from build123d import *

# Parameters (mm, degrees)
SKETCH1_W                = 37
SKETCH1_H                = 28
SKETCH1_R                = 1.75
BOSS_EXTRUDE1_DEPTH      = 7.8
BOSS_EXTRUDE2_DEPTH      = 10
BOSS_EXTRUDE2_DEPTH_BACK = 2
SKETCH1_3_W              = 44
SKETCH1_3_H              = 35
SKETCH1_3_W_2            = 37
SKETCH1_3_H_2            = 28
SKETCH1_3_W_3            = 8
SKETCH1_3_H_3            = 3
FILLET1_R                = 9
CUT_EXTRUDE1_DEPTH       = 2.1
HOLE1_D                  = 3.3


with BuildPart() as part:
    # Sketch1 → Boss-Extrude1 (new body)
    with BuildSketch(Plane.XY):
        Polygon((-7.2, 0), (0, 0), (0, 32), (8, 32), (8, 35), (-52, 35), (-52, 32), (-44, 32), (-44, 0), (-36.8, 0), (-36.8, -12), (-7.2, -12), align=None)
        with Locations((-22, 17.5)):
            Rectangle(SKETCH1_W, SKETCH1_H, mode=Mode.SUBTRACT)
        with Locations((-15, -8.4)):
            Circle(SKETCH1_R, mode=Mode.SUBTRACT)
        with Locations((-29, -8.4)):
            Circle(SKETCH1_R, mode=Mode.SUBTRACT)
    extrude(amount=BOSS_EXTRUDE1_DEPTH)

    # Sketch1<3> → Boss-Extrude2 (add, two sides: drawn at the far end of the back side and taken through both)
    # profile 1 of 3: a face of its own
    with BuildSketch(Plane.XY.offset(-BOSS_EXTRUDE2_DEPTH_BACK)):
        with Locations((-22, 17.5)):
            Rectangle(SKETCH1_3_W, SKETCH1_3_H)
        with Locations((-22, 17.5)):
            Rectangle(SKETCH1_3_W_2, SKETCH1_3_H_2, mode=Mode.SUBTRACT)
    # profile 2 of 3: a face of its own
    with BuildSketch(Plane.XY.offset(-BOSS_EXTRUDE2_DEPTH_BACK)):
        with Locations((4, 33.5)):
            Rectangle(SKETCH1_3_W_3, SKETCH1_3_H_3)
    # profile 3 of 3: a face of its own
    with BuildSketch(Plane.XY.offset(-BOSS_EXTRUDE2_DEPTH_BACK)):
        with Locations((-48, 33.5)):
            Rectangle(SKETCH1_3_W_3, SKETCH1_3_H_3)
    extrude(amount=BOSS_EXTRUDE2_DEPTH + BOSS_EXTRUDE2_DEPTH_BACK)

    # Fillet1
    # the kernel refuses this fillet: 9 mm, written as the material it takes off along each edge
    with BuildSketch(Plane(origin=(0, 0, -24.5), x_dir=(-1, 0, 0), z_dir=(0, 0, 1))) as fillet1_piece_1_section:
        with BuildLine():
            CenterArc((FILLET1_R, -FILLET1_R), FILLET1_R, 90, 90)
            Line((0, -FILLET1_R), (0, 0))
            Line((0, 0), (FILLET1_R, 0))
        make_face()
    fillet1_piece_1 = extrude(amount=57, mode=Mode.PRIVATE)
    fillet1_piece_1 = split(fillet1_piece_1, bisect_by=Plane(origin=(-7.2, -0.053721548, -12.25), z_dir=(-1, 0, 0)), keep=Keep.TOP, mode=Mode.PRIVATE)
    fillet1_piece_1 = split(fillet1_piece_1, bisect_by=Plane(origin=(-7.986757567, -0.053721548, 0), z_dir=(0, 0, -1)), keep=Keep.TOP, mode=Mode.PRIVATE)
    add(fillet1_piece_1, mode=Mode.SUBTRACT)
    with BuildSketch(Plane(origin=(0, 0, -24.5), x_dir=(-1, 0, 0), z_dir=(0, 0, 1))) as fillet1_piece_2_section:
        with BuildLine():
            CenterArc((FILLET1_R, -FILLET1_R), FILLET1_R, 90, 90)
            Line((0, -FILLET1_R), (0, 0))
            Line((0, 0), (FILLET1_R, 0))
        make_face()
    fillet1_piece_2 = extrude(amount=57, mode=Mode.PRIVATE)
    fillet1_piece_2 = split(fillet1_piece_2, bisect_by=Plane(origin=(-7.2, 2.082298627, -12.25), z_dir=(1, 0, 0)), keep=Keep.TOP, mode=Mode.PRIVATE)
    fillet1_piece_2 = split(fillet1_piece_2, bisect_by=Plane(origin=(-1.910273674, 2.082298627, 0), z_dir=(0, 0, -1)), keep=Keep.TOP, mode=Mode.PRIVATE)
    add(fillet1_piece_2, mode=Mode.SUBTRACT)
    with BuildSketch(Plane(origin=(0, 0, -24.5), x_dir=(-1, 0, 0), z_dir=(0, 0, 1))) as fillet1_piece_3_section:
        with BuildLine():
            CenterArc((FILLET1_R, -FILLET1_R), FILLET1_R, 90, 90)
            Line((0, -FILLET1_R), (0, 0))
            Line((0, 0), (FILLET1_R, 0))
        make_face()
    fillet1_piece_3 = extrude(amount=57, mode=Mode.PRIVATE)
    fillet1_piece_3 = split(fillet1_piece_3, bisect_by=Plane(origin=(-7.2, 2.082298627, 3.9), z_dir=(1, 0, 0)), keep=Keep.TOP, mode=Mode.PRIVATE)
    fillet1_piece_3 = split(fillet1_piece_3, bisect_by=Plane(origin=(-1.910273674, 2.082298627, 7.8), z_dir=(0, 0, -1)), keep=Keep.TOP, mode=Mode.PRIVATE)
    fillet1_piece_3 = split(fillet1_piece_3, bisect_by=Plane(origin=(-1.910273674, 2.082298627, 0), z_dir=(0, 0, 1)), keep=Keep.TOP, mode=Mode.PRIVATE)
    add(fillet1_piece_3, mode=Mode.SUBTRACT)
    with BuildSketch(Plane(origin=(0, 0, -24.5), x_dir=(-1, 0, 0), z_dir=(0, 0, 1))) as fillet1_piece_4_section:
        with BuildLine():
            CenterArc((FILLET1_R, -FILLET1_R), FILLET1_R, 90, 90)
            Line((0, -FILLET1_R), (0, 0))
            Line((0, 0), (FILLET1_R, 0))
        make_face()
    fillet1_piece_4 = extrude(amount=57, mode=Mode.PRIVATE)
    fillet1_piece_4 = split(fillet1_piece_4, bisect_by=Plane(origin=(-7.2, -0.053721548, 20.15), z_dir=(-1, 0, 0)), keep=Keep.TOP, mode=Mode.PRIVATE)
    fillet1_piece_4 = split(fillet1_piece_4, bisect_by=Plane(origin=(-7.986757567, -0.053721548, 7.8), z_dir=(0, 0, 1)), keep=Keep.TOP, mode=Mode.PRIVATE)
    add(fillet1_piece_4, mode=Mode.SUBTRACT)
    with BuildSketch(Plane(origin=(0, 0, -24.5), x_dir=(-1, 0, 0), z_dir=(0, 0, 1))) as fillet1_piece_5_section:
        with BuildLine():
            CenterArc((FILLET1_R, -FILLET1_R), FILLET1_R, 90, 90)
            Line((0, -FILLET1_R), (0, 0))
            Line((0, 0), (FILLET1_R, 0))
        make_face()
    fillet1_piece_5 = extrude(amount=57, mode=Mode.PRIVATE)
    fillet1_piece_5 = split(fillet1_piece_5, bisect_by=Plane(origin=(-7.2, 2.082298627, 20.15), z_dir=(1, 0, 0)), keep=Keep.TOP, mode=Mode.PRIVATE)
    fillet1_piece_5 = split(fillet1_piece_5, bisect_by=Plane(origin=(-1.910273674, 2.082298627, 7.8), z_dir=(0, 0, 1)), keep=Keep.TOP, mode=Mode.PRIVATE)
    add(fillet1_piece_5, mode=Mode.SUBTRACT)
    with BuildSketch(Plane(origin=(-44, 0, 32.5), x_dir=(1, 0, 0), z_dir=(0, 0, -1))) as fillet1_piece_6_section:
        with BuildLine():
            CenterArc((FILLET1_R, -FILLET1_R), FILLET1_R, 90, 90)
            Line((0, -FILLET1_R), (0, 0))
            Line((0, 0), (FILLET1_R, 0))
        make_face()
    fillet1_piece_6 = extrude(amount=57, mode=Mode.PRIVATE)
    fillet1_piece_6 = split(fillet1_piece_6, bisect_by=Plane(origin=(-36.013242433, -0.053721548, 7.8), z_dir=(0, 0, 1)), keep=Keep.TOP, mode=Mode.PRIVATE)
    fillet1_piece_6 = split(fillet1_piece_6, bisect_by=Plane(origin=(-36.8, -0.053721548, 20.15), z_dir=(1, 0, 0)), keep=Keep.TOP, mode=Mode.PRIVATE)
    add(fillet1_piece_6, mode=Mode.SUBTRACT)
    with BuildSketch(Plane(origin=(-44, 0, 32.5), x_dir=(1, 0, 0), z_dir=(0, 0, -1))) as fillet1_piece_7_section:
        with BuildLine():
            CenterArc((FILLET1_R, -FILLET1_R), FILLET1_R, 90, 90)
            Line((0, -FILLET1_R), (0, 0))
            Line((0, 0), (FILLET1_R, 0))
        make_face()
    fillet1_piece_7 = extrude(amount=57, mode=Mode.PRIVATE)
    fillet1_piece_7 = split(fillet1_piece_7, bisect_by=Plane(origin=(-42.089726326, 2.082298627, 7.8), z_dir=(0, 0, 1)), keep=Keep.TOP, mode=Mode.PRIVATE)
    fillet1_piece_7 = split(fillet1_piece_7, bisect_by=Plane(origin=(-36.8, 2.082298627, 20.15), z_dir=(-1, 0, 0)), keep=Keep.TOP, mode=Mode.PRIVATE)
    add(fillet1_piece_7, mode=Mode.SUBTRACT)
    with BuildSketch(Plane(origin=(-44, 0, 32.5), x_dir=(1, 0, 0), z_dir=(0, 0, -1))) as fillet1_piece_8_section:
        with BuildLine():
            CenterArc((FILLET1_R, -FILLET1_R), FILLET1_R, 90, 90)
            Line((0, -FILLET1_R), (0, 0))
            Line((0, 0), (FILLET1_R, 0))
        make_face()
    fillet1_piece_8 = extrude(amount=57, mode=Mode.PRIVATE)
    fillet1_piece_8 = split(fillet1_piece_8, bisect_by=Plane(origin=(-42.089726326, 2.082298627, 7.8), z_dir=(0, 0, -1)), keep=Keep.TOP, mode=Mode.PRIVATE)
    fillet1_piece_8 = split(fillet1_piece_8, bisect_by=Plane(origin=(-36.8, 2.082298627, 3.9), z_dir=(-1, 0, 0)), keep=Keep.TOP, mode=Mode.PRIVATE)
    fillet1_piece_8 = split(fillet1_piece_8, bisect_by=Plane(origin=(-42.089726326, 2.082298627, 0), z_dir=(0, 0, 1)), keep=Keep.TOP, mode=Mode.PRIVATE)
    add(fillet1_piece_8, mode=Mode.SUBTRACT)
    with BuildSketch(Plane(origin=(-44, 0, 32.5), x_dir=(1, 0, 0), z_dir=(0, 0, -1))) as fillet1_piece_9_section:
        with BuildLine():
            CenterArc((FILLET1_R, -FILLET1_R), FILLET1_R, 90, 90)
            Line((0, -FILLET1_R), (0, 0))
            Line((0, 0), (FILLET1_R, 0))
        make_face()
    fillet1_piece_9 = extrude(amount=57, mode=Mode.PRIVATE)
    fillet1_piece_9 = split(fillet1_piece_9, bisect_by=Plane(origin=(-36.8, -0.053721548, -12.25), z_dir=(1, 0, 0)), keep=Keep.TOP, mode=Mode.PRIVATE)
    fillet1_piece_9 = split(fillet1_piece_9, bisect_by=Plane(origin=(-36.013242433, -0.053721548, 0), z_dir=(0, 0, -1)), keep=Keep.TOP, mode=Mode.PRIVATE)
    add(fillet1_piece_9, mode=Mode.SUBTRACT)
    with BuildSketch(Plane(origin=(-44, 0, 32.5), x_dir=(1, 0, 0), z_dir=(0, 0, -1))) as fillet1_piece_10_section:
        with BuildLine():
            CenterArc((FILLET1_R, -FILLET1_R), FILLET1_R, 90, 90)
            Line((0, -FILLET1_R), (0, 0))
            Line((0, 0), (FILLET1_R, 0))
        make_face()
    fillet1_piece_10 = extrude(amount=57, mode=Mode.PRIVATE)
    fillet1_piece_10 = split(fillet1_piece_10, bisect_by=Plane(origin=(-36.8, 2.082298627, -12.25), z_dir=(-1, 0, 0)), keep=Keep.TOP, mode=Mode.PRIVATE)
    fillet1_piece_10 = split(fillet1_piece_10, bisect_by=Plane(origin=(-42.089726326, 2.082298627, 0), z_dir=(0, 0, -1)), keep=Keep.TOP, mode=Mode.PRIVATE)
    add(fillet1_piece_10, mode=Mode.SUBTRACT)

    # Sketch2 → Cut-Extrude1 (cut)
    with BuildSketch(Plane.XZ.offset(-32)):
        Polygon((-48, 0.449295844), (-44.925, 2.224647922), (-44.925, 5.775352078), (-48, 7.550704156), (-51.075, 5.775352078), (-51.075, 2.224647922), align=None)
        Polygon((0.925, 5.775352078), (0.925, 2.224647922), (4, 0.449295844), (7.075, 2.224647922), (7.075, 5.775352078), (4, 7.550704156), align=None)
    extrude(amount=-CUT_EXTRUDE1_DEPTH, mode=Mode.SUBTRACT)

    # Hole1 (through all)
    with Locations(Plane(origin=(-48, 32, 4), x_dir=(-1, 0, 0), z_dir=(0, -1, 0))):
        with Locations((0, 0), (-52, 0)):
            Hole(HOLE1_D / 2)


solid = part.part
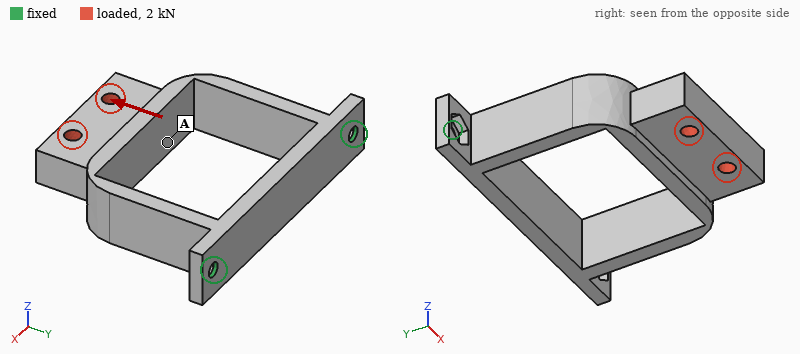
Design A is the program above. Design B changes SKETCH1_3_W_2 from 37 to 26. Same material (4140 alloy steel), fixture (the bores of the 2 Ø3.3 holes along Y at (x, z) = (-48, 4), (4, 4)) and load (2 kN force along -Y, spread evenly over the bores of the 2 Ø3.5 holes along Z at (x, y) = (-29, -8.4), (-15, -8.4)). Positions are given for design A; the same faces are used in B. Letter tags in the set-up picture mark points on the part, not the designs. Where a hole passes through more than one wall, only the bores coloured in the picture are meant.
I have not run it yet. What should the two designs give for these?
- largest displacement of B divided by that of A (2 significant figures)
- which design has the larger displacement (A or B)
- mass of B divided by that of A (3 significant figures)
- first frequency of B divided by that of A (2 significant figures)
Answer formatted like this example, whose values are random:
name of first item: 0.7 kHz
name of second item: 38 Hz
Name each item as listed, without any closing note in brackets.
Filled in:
largest displacement of B divided by that of A: 0.52
which design has the larger displacement: A
mass of B divided by that of A: 1.43
first frequency of B divided by that of A: 0.93
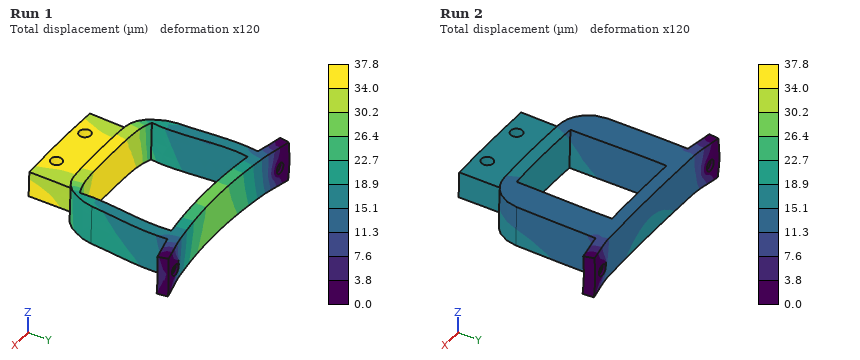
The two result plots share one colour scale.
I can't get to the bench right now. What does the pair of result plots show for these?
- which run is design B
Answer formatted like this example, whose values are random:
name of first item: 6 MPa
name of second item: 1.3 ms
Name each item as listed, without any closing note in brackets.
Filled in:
which run is design B: Run 2
